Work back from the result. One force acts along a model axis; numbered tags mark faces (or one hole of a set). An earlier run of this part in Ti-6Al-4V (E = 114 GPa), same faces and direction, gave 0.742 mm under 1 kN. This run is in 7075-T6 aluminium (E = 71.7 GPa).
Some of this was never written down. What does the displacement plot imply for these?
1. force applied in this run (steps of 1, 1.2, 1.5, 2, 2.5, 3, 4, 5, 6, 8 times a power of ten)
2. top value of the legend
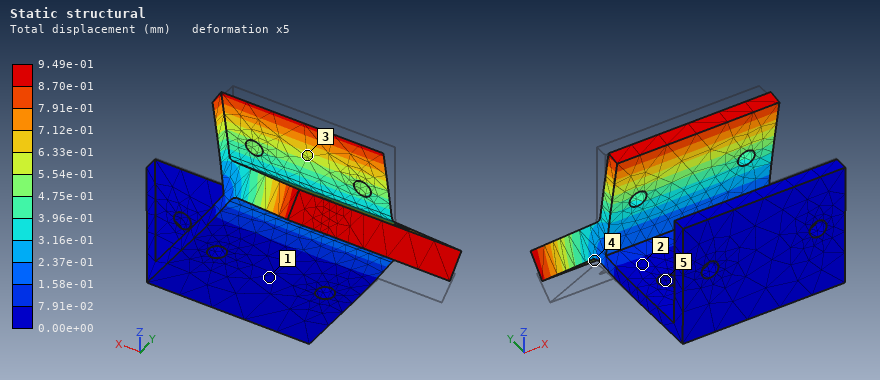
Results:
800 N
9.49e-01 mm
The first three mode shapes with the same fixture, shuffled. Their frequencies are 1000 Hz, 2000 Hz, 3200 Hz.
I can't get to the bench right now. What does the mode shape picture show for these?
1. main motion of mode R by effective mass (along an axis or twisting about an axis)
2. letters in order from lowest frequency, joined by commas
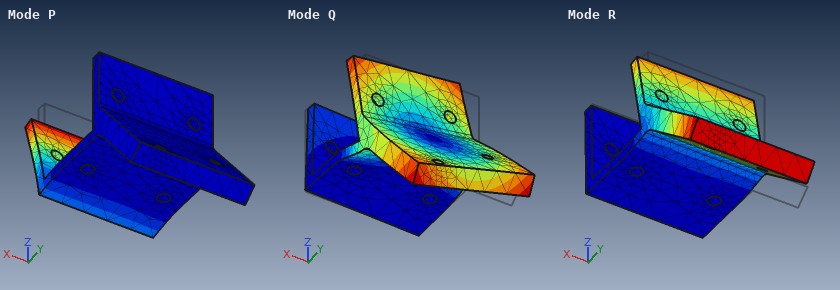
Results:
along Z
R, P, Q
